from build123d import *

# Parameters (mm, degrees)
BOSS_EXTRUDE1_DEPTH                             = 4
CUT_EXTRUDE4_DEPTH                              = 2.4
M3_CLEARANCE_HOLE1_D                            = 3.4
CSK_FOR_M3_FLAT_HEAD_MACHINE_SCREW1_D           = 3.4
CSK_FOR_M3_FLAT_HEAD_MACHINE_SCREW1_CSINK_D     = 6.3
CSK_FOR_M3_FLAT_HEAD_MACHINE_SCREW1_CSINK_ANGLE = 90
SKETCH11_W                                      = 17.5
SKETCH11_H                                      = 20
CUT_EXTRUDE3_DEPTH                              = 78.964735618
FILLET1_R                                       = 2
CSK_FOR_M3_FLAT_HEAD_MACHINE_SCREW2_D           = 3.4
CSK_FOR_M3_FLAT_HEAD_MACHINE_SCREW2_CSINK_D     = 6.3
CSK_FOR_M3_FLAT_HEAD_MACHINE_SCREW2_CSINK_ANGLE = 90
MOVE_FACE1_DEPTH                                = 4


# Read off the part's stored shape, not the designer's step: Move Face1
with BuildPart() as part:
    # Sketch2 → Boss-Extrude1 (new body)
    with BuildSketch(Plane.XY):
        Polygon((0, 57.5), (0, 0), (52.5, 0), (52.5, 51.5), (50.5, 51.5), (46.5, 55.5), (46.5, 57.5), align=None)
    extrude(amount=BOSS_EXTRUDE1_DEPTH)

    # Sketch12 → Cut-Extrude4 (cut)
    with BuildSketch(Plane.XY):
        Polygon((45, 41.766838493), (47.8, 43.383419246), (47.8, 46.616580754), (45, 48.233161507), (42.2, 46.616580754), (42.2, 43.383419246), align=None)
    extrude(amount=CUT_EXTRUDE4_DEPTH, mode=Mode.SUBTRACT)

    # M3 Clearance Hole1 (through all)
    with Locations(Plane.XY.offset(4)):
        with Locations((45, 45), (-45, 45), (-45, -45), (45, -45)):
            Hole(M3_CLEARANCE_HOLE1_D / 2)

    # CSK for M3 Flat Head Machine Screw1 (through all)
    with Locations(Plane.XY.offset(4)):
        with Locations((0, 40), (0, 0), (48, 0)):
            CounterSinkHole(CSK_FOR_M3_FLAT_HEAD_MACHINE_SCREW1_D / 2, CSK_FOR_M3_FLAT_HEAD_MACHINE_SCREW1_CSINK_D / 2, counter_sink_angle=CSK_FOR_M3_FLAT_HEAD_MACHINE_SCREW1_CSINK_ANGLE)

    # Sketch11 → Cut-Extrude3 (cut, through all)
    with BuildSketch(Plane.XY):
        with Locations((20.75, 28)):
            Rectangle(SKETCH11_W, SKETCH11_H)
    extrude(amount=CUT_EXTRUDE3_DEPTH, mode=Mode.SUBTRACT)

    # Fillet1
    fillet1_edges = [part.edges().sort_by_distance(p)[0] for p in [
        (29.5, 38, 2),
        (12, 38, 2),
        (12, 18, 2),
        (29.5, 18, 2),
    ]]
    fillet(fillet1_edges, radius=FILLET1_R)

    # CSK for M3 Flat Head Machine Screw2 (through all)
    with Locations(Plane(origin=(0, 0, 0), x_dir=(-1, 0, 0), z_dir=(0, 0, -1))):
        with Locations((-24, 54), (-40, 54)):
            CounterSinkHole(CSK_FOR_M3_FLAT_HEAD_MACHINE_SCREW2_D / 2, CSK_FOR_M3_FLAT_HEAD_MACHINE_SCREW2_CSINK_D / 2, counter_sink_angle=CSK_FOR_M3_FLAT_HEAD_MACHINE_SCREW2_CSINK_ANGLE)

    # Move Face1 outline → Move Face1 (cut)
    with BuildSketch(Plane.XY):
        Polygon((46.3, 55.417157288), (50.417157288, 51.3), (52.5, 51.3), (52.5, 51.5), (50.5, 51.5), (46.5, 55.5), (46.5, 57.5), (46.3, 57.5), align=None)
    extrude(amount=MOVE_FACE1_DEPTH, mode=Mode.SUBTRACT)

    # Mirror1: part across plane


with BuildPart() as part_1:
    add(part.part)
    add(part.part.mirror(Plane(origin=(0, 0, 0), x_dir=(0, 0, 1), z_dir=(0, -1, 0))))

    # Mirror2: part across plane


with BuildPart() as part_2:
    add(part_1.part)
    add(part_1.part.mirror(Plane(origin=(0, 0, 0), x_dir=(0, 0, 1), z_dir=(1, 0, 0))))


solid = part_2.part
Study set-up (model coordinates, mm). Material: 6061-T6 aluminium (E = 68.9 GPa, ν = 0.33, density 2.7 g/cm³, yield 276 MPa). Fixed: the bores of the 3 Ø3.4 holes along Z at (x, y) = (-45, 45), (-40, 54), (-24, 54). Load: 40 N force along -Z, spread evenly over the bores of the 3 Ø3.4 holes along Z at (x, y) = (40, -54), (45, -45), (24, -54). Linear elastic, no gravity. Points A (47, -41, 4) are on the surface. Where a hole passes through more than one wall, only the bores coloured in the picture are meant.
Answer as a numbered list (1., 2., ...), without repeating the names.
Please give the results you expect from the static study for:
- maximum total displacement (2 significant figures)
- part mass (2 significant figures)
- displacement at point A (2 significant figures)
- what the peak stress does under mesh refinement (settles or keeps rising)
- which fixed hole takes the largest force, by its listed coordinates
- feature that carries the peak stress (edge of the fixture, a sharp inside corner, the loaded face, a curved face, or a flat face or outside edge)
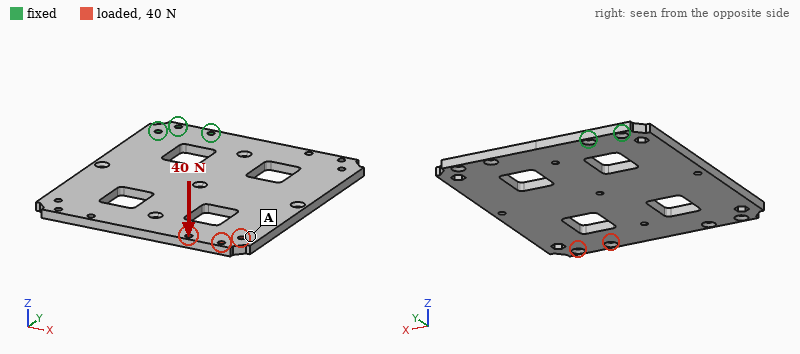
1. 1.6 mm
2. 110 g
3. 1.3 mm
4. keeps rising
5. (-40, 54)
6. edge of the fixture
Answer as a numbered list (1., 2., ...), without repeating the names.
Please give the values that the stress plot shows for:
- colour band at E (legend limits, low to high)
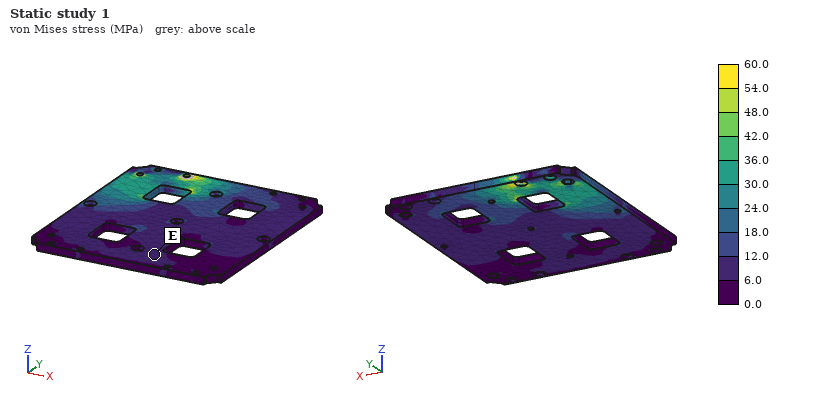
1. 6.0 to 12.0 MPa
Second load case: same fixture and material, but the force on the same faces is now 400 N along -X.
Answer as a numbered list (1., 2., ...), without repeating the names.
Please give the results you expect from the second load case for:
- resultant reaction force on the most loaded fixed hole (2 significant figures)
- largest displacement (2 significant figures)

1. 1.6 kN
2. 0.17 mm
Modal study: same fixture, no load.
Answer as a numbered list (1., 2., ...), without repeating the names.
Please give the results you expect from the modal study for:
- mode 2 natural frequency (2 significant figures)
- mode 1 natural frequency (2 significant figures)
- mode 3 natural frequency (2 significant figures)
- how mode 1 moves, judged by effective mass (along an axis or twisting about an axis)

1. 390 Hz
2. 170 Hz
3. 900 Hz
4. along Z
